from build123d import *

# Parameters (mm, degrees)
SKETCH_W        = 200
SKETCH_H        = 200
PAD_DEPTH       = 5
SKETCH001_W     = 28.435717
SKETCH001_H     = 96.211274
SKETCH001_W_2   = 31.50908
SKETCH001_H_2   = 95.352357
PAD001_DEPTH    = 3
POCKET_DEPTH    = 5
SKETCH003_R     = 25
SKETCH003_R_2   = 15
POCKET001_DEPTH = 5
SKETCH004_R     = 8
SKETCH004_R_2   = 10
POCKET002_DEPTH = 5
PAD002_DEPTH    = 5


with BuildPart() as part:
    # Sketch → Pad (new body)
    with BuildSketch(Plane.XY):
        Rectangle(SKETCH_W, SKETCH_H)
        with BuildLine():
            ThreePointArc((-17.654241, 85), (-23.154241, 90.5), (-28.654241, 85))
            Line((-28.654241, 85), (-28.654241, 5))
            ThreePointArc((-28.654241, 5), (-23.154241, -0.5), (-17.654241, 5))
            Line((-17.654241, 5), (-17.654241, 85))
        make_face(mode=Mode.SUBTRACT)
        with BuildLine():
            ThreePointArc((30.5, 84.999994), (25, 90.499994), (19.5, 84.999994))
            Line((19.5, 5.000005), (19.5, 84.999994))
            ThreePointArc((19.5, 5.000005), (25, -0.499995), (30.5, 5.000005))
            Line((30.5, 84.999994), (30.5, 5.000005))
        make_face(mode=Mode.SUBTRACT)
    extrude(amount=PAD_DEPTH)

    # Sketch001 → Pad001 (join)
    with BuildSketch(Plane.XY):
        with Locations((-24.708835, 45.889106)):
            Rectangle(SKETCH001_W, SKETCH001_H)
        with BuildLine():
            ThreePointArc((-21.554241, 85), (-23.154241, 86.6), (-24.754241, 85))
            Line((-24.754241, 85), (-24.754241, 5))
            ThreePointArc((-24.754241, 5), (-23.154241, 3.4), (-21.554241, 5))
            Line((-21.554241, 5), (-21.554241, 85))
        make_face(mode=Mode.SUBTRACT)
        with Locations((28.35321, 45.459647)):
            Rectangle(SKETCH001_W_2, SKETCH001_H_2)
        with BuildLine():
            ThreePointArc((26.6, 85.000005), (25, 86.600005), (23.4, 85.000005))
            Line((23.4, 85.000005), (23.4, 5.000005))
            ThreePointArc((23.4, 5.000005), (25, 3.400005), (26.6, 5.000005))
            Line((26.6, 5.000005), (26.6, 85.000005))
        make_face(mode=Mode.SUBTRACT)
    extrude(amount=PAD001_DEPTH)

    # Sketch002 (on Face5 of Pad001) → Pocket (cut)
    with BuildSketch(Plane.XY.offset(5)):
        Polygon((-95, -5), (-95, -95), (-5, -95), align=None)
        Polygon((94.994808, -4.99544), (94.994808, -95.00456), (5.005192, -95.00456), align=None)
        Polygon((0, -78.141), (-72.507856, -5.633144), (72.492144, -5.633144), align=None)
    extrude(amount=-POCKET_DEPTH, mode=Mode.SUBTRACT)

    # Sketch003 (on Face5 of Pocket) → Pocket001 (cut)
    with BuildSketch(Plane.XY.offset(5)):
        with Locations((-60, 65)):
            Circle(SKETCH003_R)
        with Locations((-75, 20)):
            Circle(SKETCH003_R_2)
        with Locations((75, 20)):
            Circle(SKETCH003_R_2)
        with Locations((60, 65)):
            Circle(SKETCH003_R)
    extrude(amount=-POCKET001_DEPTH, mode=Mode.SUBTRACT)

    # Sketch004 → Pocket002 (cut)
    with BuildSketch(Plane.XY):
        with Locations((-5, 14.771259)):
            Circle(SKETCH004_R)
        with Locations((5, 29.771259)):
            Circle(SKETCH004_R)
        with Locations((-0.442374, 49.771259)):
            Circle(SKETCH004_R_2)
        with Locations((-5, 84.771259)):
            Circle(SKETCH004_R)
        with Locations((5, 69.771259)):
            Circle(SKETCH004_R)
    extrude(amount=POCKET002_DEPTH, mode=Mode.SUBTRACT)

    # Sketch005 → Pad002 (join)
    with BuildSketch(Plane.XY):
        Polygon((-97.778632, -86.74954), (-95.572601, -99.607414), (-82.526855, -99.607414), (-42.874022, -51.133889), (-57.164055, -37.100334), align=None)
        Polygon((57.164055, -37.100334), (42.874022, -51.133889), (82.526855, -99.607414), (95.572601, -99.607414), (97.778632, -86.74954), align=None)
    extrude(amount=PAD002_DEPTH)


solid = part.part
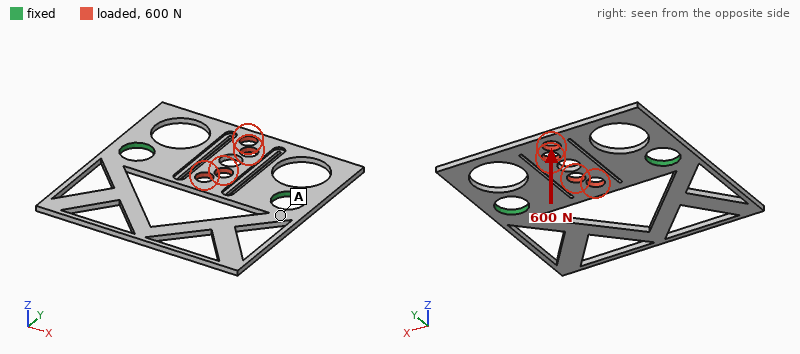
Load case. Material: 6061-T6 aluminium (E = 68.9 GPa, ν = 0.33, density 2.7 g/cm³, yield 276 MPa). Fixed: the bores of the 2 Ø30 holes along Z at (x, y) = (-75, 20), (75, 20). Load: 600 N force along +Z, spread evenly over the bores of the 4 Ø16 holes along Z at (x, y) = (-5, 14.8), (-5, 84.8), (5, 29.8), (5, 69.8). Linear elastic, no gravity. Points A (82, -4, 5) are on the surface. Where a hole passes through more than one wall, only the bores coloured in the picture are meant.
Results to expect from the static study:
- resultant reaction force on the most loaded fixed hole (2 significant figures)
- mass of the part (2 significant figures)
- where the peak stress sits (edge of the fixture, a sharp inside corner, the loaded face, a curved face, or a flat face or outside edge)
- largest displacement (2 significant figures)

320 N
290 g
a curved face
0.89 mm
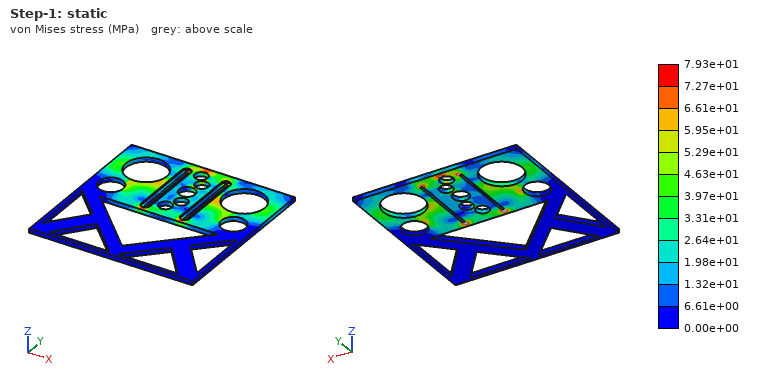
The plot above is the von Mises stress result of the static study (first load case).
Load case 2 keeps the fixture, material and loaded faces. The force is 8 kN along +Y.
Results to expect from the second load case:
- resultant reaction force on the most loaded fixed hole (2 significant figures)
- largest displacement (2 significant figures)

4.1 kN
0.15 mm
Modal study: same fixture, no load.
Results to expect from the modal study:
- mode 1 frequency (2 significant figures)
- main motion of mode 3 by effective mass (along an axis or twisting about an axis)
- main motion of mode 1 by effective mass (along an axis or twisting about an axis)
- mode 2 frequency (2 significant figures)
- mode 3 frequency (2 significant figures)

230 Hz
along Z
along Z
400 Hz
530 Hz
